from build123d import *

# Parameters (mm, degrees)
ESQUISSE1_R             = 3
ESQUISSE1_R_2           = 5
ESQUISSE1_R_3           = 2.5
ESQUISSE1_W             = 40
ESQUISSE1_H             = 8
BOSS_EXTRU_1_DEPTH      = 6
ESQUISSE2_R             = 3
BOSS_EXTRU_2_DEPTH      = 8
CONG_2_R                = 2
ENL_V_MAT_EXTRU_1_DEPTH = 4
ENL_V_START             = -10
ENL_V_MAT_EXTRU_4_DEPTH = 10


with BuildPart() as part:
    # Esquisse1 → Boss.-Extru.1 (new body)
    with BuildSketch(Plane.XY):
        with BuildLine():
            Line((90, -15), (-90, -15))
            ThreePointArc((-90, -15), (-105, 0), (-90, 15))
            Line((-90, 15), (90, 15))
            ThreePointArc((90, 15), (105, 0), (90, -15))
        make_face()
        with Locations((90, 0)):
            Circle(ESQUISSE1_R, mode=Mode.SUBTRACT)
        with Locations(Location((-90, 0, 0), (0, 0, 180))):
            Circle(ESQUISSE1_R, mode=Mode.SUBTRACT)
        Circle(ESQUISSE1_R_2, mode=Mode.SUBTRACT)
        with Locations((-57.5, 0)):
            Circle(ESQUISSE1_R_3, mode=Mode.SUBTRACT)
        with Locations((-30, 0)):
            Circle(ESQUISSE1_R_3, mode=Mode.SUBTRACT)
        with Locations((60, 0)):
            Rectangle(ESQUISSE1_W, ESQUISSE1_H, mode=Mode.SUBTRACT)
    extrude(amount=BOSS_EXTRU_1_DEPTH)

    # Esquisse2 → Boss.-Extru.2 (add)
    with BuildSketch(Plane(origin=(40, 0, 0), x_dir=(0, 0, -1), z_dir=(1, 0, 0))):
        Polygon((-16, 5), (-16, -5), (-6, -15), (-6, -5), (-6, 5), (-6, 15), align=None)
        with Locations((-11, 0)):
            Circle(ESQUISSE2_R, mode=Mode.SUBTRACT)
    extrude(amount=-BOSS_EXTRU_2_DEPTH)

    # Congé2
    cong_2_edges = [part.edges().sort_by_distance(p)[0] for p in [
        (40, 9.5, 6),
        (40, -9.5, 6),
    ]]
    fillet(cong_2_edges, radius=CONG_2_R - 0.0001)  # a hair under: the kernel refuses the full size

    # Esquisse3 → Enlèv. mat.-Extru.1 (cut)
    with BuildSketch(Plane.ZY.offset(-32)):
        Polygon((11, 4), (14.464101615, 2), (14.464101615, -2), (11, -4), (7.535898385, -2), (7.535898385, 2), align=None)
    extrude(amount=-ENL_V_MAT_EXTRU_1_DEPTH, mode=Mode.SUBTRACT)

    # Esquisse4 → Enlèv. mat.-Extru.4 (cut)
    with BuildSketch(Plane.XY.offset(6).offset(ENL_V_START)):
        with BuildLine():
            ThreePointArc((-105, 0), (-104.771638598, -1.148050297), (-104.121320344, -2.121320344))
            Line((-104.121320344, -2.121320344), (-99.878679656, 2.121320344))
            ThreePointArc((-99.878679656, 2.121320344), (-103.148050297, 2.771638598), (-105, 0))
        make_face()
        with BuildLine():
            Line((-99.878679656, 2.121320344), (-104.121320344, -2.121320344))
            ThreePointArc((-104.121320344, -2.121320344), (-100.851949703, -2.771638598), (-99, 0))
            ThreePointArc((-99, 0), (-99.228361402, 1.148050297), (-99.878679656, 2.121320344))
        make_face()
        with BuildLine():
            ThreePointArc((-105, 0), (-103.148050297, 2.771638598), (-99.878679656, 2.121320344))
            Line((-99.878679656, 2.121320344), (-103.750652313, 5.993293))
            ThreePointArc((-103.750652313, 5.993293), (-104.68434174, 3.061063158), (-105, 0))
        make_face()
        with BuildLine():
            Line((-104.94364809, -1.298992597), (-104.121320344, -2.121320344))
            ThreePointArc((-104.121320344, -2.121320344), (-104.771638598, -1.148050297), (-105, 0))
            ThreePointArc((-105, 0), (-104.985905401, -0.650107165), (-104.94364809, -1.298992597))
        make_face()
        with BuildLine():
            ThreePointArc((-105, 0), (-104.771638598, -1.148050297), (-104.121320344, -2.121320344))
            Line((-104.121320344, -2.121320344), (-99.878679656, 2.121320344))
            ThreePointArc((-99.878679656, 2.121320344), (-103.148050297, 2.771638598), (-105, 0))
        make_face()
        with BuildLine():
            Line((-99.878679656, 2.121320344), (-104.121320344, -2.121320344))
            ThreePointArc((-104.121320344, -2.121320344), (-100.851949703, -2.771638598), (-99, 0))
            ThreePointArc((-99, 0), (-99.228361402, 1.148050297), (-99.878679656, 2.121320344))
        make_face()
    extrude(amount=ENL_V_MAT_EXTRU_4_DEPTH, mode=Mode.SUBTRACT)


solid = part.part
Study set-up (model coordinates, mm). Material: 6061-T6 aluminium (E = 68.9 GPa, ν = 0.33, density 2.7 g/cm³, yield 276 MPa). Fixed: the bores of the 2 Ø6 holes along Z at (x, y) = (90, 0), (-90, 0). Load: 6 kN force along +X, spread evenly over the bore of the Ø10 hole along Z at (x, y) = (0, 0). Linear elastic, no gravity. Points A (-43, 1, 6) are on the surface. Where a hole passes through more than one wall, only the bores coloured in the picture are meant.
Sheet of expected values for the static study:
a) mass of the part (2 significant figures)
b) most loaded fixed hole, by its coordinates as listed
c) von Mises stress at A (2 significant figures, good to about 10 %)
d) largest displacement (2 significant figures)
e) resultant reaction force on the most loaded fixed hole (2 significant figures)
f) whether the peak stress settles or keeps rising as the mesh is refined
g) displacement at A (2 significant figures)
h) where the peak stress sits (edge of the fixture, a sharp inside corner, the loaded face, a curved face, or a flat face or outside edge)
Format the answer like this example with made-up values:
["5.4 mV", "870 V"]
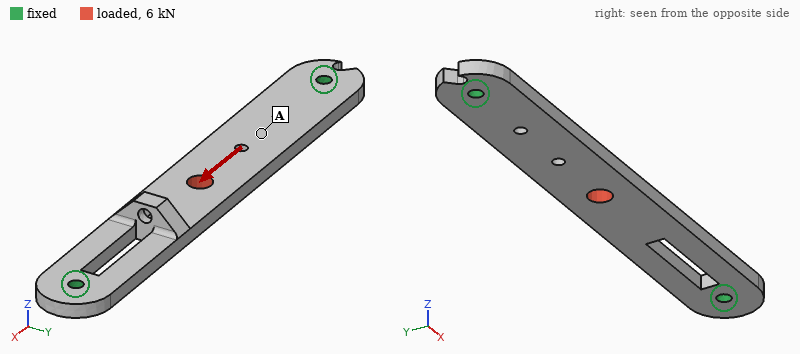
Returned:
["94 g", "(-90, 0)", "15 MPa", "29 µm", "3.2 kN", "keeps rising", "15 µm", "edge of the fixture"]
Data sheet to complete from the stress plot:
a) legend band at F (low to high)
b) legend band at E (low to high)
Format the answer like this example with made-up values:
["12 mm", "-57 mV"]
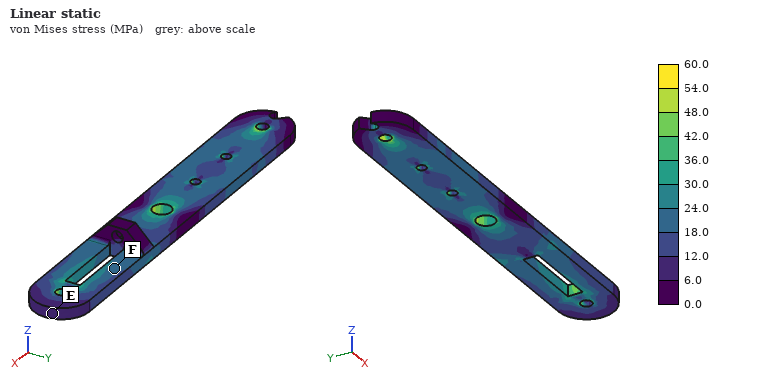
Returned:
["18.0 to 24.0 MPa", "6.0 to 12.0 MPa"]
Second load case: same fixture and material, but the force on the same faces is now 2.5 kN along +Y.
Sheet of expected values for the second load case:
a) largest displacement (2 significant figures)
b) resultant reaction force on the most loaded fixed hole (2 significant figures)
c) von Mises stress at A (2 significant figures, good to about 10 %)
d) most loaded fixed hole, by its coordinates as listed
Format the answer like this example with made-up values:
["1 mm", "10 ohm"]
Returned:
["0.25 mm", "1.3 kN", "21 MPa", "(-90, 0)"]
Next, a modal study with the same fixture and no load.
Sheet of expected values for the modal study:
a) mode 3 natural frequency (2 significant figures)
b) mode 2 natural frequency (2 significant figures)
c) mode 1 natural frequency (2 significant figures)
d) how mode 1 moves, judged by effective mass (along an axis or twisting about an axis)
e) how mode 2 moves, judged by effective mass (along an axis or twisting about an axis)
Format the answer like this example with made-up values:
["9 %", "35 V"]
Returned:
["2500 Hz", "2400 Hz", "910 Hz", "along Z", "along Y"]
